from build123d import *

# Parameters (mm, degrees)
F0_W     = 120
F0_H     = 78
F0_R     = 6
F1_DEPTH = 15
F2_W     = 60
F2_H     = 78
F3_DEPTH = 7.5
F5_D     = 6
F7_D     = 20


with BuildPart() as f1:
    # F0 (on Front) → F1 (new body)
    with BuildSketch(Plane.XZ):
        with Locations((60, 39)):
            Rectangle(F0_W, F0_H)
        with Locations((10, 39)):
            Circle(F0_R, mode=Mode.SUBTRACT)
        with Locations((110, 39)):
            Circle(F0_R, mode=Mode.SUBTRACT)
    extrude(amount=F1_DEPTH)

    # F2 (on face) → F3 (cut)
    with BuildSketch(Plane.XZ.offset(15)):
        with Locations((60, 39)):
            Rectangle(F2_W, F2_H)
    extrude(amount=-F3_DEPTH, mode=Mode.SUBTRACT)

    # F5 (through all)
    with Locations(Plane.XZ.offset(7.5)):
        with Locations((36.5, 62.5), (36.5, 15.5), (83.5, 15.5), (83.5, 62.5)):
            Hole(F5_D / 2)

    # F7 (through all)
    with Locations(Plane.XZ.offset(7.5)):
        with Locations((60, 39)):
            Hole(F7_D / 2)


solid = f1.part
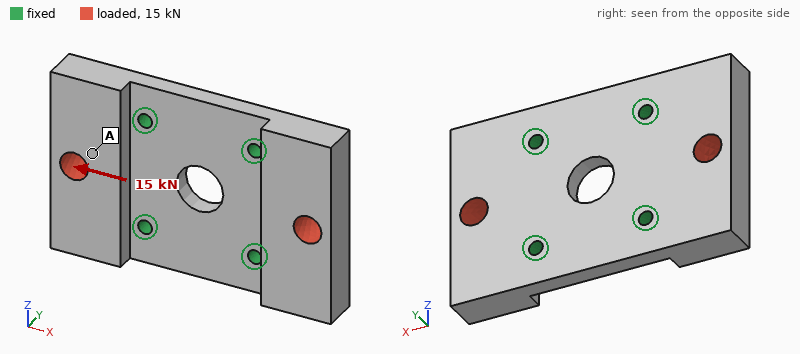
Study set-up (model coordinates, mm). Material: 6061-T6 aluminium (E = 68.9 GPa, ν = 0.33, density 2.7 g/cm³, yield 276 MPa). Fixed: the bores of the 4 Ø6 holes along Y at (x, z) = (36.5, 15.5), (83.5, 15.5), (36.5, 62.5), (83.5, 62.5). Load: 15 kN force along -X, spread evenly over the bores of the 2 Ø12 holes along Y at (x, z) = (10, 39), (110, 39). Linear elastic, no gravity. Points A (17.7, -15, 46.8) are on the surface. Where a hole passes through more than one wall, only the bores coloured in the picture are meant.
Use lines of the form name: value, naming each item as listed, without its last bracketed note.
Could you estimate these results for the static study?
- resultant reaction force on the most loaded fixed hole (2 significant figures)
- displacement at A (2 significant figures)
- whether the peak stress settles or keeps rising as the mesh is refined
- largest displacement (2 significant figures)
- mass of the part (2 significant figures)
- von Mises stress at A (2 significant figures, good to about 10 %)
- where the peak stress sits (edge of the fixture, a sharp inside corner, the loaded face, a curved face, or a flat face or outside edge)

resultant reaction force on the most loaded fixed hole: 3.9 kN
displacement at A: 36 µm
whether the peak stress settles or keeps rising as the mesh is refined: keeps rising
largest displacement: 64 µm
mass of the part: 270 g
von Mises stress at A: 17 MPa
where the peak stress sits: edge of the fixture
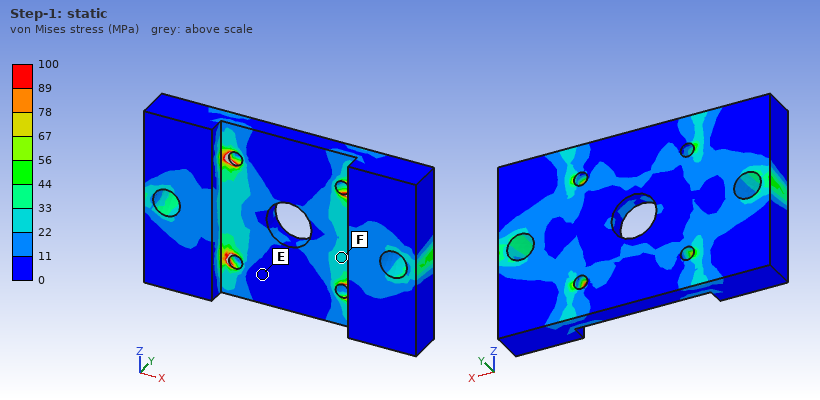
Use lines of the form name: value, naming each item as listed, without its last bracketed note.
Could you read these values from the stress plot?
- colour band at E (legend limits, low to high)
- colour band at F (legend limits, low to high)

colour band at E: 0 to 11 MPa
colour band at F: 22 to 33 MPa
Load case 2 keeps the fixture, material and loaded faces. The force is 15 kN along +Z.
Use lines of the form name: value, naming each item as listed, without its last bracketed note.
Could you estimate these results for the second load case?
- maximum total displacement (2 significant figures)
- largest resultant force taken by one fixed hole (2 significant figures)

maximum total displacement: 22 µm
largest resultant force taken by one fixed hole: 4.6 kN
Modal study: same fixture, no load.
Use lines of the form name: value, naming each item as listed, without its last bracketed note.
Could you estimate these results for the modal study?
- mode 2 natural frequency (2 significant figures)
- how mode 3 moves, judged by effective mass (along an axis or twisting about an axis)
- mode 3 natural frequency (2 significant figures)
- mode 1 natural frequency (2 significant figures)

mode 2 natural frequency: 3400 Hz
how mode 3 moves, judged by effective mass: twisting about X
mode 3 natural frequency: 6600 Hz
mode 1 natural frequency: 3300 Hz
